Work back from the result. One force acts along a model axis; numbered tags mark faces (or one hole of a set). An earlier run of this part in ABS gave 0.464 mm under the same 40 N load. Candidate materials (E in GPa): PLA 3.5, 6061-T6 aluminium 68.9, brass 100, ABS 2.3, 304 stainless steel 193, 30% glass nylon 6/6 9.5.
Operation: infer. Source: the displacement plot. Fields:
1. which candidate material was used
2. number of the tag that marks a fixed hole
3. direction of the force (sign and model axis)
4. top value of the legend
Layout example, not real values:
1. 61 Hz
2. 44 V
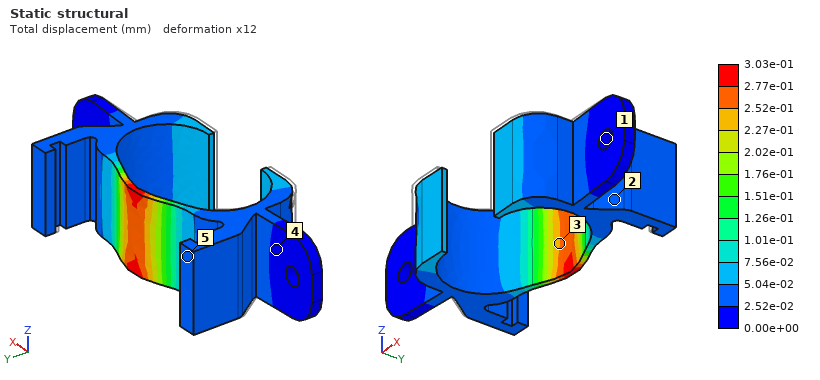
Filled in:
1. PLA
2. 1
3. +Y
4. 3.03e-01 mm
